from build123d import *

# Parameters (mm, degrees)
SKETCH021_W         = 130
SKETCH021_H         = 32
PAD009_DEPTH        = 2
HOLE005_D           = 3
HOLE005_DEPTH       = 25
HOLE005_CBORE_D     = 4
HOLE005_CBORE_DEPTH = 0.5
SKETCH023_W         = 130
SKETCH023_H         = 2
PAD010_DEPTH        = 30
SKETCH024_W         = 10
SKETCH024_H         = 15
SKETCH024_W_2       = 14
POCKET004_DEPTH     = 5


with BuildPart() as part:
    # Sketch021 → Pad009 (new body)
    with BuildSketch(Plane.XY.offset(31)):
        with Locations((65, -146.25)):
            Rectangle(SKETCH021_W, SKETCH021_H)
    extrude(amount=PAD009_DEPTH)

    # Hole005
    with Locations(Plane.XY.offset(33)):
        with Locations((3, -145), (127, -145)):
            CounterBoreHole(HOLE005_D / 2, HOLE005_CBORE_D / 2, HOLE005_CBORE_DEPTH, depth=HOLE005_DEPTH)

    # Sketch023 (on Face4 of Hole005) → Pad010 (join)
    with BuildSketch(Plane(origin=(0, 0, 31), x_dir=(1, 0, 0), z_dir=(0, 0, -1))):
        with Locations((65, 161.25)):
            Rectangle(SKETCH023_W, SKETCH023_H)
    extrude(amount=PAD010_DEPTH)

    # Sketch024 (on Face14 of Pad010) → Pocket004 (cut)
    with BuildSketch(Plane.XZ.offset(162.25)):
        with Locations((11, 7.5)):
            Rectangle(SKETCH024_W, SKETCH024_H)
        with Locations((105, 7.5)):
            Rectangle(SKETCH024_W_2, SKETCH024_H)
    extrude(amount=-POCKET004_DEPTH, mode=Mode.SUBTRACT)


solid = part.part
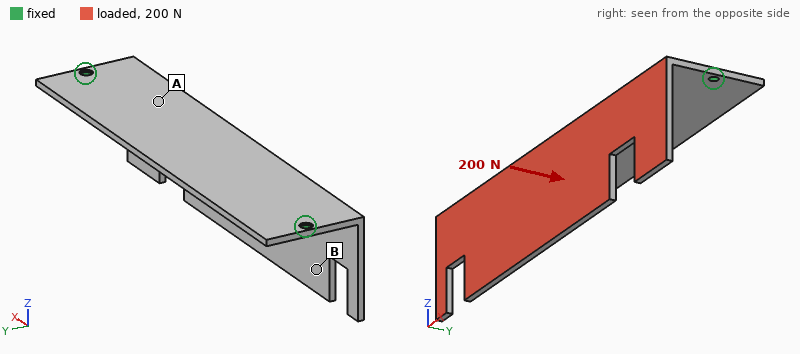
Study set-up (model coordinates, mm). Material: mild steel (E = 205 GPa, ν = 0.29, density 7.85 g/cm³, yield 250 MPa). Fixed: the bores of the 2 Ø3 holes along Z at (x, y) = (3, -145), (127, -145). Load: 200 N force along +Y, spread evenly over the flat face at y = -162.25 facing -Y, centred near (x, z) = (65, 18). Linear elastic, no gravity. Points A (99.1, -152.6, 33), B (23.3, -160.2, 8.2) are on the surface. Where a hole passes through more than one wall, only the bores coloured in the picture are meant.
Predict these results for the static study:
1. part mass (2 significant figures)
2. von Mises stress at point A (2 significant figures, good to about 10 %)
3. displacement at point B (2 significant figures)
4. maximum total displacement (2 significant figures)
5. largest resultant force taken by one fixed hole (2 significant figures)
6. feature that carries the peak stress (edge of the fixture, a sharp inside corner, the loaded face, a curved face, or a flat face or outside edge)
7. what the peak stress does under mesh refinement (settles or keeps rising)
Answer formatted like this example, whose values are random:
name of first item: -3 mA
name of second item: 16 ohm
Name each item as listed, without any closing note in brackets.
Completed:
part mass: 120 g
von Mises stress at point A: 28 MPa
displacement at point B: 0.20 mm
maximum total displacement: 0.29 mm
largest resultant force taken by one fixed hole: 100 N
feature that carries the peak stress: edge of the fixture
what the peak stress does under mesh refinement: keeps rising
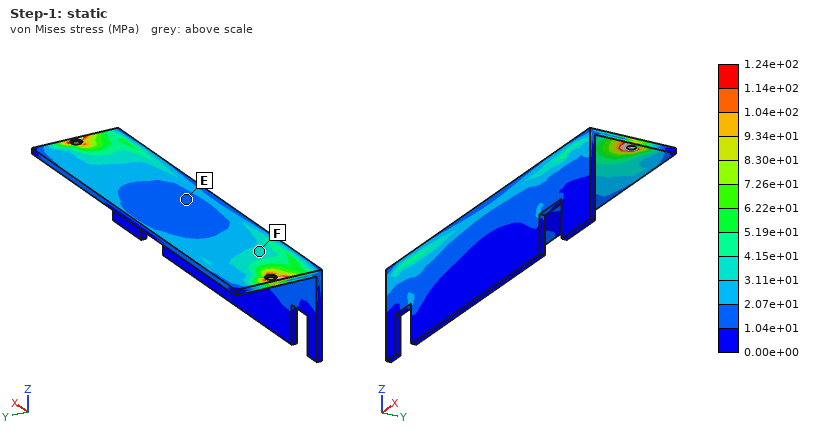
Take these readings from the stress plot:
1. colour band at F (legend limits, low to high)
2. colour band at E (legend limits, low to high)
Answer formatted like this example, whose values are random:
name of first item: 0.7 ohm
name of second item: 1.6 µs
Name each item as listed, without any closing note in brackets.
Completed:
colour band at F: 3.11e+01 to 4.15e+01 MPa
colour band at E: 1.04e+01 to 2.07e+01 MPa
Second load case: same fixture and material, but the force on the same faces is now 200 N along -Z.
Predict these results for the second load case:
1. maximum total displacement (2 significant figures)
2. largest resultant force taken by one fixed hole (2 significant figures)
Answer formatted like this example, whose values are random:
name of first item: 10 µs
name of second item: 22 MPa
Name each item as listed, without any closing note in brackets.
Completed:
maximum total displacement: 0.20 mm
largest resultant force taken by one fixed hole: 100 N
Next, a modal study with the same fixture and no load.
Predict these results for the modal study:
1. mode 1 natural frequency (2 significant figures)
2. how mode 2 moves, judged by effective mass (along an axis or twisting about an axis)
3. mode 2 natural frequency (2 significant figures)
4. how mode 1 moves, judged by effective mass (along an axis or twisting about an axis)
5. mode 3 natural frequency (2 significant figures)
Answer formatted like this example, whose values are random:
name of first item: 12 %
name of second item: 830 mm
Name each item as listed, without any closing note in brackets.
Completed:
mode 1 natural frequency: 590 Hz
how mode 2 moves, judged by effective mass: along Z
mode 2 natural frequency: 1100 Hz
how mode 1 moves, judged by effective mass: along Y
mode 3 natural frequency: 1200 Hz
